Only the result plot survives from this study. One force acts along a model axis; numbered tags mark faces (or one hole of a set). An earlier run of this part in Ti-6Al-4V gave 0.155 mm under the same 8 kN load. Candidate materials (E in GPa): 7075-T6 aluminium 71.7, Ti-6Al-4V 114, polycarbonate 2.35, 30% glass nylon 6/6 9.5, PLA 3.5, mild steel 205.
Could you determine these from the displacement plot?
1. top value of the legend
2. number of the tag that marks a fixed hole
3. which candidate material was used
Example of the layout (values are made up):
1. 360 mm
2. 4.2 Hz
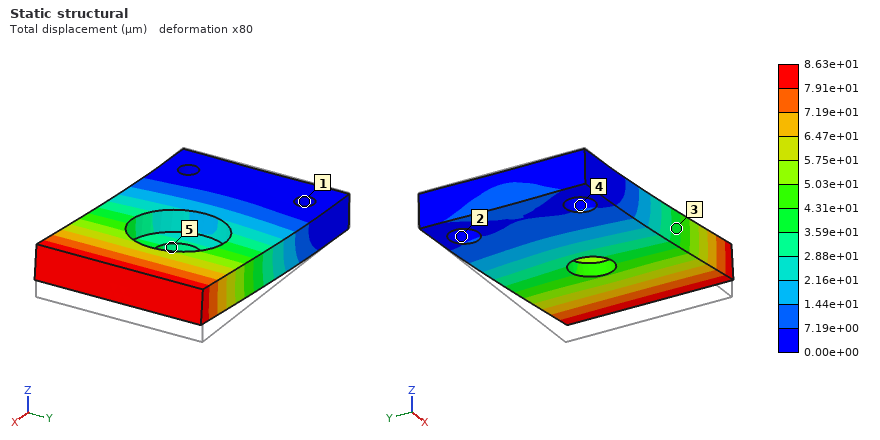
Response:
1. 8.63e+01 µm
2. 1
3. mild steel
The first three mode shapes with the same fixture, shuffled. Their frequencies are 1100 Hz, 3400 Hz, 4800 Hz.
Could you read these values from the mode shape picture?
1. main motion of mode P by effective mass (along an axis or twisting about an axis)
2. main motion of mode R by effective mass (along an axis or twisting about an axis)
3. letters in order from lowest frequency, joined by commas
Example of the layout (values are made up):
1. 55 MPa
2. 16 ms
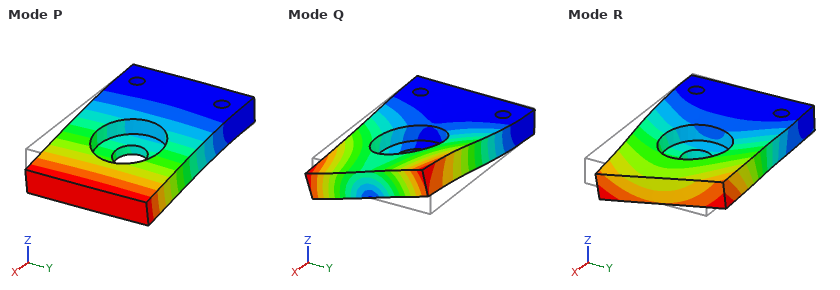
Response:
1. along Z
2. along Y
3. P, Q, R
